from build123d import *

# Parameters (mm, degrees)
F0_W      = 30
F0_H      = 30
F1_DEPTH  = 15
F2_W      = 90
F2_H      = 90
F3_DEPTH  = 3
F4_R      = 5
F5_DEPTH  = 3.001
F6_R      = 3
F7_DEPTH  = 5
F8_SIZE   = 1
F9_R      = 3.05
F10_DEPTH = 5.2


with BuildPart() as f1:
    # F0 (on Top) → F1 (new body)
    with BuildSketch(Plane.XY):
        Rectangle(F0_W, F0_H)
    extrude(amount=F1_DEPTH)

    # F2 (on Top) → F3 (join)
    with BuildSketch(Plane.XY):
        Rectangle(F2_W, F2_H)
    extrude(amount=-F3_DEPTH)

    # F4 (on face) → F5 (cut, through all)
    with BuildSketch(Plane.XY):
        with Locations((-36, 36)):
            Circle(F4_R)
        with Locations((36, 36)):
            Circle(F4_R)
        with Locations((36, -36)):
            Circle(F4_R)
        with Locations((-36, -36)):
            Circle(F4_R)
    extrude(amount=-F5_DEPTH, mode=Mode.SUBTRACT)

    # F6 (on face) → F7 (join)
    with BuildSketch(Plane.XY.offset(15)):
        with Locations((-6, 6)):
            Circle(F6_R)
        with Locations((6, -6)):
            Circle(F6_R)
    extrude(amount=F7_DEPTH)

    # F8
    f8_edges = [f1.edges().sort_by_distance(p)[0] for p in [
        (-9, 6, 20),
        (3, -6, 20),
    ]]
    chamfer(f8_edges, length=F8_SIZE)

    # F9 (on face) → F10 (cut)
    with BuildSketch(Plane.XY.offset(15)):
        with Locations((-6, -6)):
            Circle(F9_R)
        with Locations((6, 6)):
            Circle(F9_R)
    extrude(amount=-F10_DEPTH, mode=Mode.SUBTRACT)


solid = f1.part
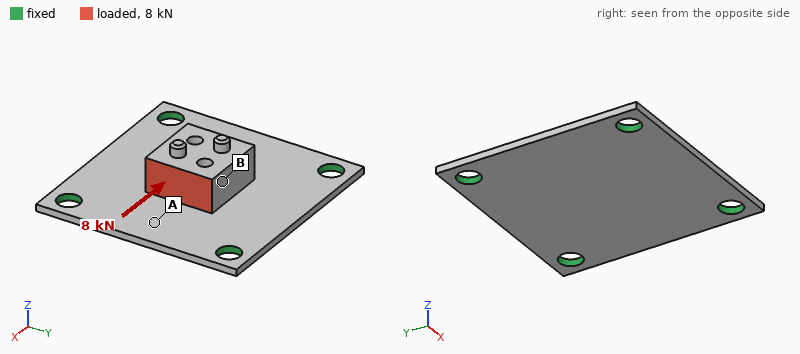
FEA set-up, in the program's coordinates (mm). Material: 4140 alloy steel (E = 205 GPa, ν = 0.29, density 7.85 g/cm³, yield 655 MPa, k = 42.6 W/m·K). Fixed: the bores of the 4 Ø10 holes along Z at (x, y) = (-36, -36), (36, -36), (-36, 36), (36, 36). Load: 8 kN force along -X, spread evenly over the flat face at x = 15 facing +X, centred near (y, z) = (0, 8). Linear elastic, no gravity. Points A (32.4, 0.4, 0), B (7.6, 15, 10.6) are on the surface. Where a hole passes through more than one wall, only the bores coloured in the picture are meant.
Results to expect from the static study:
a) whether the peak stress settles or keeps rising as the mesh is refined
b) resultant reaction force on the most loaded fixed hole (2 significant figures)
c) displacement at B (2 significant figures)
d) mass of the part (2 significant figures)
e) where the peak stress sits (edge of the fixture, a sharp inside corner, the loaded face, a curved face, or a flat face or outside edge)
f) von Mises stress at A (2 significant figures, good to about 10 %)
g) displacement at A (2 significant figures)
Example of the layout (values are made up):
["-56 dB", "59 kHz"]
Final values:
["keeps rising", "2.4 kN", "0.066 mm", "290 g", "edge of the fixture", "63 MPa", "0.070 mm"]
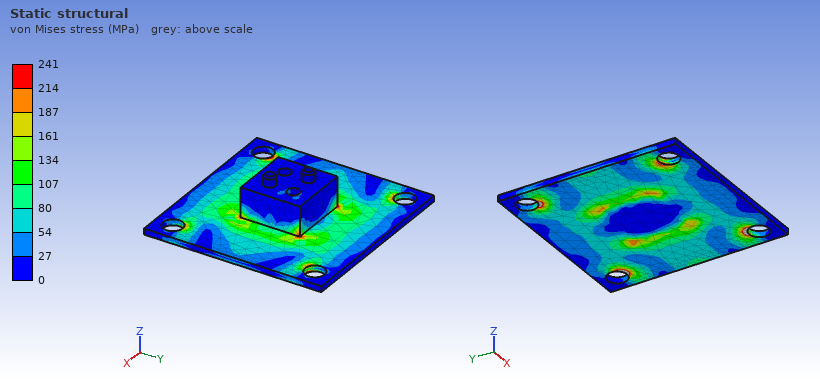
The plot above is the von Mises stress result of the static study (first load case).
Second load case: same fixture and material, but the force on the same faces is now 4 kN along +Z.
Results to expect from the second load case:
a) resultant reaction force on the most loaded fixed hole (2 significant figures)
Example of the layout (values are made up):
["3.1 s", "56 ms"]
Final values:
["1.6 kN"]
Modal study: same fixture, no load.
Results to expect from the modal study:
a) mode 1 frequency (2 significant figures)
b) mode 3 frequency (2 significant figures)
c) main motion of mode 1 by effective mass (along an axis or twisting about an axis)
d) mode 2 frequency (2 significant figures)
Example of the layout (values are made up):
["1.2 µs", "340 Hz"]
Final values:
["1900 Hz", "3400 Hz", "along Z", "3400 Hz"]
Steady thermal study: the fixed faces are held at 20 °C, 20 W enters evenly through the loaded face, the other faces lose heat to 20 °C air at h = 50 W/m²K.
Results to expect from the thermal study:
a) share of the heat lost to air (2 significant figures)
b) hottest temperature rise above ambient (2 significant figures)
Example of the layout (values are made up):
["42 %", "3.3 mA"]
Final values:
["54 %", "37 K"]
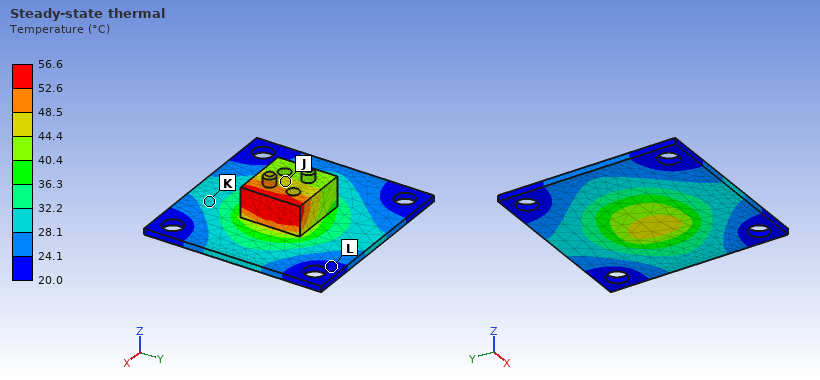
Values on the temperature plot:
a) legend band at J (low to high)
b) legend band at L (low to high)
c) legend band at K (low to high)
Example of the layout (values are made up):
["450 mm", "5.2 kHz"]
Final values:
["44.4 to 48.5 °C", "20.0 to 24.1 °C", "28.1 to 32.2 °C"]
